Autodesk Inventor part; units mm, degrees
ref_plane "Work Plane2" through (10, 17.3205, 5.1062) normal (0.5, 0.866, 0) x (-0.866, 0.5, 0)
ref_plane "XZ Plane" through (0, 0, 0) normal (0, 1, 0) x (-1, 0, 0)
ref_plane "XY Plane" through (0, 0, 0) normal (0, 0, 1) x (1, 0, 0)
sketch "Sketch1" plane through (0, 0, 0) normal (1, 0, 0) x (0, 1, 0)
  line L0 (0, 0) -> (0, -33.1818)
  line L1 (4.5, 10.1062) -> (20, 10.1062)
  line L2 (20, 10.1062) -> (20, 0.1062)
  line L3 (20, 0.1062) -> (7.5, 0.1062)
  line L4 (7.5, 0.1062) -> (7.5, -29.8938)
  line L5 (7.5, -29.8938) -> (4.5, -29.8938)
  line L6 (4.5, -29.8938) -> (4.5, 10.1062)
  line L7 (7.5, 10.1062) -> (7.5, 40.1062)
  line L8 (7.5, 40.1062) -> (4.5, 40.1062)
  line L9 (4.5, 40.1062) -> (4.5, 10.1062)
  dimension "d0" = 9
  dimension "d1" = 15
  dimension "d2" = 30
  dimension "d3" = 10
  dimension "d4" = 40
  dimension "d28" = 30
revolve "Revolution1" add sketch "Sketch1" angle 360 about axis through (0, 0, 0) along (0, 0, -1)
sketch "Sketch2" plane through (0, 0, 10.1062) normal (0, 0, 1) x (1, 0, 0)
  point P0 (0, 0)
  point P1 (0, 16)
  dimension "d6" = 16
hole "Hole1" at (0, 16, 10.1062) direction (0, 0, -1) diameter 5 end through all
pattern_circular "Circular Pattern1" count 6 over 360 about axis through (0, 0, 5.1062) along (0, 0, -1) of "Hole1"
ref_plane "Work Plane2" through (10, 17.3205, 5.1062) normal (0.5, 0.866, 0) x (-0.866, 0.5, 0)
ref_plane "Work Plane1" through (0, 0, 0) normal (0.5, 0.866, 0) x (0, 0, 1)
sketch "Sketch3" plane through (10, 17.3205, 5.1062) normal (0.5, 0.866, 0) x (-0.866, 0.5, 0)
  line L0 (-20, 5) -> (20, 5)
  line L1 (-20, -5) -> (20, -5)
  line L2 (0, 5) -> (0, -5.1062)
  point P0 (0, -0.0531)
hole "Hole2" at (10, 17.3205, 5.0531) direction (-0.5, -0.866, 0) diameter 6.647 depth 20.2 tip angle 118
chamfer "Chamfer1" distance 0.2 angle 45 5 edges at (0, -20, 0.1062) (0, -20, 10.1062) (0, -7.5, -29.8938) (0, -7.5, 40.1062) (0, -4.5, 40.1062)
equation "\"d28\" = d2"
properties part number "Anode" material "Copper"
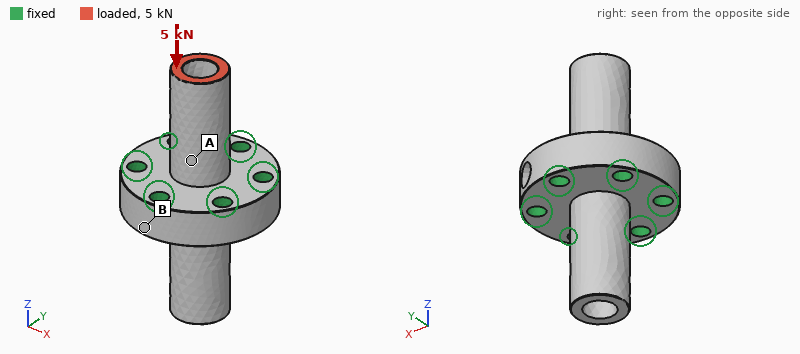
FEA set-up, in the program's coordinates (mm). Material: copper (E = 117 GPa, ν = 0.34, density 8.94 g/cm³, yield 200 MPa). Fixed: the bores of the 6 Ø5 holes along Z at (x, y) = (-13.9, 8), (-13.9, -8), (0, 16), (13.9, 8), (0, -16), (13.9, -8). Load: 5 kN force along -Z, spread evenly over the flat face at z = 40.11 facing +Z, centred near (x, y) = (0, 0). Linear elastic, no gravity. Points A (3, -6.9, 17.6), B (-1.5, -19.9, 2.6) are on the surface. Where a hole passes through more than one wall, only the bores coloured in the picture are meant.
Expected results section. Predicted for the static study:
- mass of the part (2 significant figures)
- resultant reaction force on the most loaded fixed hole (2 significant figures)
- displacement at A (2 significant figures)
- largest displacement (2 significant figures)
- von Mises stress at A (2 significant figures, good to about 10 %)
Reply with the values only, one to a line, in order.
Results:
150 g
920 N
5.7 µm
15 µm
41 MPa
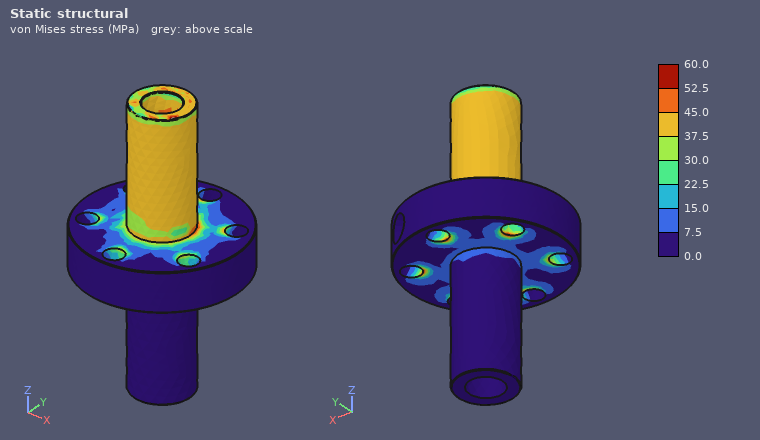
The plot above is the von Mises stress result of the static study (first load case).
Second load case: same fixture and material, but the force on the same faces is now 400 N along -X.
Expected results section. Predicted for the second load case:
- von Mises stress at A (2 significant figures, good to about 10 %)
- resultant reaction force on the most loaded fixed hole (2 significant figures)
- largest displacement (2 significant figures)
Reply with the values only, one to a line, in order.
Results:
15 MPa
380 N
26 µm
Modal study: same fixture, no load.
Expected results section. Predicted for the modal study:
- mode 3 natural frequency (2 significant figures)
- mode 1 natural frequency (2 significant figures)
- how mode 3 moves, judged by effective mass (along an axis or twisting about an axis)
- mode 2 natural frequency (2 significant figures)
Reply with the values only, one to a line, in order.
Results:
6900 Hz
6200 Hz
along Y
6200 Hz
